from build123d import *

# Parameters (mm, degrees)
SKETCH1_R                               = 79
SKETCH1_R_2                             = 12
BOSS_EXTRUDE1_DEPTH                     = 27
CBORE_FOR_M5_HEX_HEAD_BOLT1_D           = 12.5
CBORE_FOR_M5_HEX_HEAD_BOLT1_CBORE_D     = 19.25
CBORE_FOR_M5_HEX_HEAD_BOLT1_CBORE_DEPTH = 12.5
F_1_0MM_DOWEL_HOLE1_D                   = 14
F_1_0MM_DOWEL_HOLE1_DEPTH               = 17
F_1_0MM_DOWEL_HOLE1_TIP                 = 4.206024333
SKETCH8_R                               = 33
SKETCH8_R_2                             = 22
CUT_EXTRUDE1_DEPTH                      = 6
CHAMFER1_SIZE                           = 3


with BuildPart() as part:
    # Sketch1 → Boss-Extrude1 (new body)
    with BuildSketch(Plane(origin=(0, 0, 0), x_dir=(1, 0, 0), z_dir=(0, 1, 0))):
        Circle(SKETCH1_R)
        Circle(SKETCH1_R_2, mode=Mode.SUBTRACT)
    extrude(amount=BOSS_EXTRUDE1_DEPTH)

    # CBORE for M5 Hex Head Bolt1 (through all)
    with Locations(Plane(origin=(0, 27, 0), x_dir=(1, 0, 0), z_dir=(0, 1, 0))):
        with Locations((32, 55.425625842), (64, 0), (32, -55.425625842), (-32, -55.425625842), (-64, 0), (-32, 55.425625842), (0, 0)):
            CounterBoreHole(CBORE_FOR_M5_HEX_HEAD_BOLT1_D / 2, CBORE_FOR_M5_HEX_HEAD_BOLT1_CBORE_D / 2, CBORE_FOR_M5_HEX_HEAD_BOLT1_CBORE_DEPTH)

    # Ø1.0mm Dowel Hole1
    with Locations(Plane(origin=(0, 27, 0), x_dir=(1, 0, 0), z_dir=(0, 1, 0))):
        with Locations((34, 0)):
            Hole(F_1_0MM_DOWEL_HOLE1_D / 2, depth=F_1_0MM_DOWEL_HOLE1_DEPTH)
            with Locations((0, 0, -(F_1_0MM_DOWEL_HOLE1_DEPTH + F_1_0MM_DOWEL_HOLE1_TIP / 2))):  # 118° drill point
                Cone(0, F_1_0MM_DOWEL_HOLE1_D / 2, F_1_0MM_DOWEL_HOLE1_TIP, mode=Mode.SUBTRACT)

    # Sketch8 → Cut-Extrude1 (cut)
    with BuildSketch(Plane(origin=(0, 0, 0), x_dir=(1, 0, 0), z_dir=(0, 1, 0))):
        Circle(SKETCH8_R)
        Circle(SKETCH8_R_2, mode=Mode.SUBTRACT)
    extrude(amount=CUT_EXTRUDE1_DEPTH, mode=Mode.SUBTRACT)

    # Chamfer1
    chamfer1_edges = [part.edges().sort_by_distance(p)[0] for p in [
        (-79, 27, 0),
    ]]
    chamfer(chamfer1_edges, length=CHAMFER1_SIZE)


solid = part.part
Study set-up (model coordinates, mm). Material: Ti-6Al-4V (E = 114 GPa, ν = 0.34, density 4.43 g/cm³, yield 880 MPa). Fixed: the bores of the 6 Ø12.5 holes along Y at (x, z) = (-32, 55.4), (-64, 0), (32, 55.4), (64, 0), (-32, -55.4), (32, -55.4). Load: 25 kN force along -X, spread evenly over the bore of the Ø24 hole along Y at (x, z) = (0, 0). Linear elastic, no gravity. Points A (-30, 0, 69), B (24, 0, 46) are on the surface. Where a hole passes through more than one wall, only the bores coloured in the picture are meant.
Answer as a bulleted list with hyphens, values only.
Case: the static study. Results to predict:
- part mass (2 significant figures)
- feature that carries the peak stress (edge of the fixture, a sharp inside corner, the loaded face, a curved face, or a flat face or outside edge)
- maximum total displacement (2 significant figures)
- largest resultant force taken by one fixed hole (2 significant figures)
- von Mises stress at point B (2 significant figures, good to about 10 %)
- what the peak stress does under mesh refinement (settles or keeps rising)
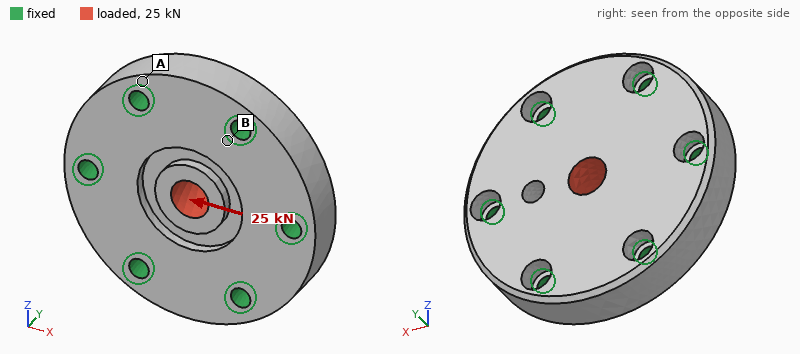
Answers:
- 2.1 kg
- a sharp inside corner
- 7.9 µm
- 6.1 kN
- 7.0 MPa
- keeps rising
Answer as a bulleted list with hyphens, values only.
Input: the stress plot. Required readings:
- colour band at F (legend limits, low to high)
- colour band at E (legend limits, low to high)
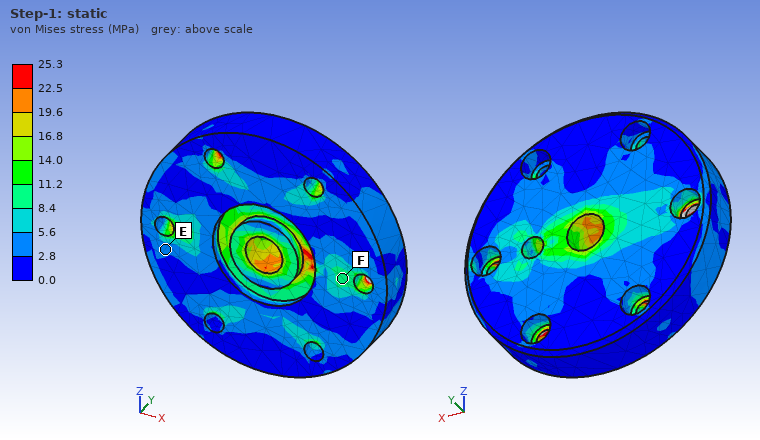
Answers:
- 8.4 to 11.2 MPa
- 2.8 to 5.6 MPa
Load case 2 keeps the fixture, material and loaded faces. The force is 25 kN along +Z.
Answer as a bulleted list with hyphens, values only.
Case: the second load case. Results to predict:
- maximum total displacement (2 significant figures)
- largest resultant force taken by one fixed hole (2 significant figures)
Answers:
- 7.4 µm
- 5.4 kN
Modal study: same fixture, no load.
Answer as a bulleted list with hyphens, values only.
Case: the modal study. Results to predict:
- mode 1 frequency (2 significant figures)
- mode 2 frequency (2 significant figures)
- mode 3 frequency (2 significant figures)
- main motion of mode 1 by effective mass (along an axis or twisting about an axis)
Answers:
- 9000 Hz
- 14 kHz
- 14 kHz
- along Y
